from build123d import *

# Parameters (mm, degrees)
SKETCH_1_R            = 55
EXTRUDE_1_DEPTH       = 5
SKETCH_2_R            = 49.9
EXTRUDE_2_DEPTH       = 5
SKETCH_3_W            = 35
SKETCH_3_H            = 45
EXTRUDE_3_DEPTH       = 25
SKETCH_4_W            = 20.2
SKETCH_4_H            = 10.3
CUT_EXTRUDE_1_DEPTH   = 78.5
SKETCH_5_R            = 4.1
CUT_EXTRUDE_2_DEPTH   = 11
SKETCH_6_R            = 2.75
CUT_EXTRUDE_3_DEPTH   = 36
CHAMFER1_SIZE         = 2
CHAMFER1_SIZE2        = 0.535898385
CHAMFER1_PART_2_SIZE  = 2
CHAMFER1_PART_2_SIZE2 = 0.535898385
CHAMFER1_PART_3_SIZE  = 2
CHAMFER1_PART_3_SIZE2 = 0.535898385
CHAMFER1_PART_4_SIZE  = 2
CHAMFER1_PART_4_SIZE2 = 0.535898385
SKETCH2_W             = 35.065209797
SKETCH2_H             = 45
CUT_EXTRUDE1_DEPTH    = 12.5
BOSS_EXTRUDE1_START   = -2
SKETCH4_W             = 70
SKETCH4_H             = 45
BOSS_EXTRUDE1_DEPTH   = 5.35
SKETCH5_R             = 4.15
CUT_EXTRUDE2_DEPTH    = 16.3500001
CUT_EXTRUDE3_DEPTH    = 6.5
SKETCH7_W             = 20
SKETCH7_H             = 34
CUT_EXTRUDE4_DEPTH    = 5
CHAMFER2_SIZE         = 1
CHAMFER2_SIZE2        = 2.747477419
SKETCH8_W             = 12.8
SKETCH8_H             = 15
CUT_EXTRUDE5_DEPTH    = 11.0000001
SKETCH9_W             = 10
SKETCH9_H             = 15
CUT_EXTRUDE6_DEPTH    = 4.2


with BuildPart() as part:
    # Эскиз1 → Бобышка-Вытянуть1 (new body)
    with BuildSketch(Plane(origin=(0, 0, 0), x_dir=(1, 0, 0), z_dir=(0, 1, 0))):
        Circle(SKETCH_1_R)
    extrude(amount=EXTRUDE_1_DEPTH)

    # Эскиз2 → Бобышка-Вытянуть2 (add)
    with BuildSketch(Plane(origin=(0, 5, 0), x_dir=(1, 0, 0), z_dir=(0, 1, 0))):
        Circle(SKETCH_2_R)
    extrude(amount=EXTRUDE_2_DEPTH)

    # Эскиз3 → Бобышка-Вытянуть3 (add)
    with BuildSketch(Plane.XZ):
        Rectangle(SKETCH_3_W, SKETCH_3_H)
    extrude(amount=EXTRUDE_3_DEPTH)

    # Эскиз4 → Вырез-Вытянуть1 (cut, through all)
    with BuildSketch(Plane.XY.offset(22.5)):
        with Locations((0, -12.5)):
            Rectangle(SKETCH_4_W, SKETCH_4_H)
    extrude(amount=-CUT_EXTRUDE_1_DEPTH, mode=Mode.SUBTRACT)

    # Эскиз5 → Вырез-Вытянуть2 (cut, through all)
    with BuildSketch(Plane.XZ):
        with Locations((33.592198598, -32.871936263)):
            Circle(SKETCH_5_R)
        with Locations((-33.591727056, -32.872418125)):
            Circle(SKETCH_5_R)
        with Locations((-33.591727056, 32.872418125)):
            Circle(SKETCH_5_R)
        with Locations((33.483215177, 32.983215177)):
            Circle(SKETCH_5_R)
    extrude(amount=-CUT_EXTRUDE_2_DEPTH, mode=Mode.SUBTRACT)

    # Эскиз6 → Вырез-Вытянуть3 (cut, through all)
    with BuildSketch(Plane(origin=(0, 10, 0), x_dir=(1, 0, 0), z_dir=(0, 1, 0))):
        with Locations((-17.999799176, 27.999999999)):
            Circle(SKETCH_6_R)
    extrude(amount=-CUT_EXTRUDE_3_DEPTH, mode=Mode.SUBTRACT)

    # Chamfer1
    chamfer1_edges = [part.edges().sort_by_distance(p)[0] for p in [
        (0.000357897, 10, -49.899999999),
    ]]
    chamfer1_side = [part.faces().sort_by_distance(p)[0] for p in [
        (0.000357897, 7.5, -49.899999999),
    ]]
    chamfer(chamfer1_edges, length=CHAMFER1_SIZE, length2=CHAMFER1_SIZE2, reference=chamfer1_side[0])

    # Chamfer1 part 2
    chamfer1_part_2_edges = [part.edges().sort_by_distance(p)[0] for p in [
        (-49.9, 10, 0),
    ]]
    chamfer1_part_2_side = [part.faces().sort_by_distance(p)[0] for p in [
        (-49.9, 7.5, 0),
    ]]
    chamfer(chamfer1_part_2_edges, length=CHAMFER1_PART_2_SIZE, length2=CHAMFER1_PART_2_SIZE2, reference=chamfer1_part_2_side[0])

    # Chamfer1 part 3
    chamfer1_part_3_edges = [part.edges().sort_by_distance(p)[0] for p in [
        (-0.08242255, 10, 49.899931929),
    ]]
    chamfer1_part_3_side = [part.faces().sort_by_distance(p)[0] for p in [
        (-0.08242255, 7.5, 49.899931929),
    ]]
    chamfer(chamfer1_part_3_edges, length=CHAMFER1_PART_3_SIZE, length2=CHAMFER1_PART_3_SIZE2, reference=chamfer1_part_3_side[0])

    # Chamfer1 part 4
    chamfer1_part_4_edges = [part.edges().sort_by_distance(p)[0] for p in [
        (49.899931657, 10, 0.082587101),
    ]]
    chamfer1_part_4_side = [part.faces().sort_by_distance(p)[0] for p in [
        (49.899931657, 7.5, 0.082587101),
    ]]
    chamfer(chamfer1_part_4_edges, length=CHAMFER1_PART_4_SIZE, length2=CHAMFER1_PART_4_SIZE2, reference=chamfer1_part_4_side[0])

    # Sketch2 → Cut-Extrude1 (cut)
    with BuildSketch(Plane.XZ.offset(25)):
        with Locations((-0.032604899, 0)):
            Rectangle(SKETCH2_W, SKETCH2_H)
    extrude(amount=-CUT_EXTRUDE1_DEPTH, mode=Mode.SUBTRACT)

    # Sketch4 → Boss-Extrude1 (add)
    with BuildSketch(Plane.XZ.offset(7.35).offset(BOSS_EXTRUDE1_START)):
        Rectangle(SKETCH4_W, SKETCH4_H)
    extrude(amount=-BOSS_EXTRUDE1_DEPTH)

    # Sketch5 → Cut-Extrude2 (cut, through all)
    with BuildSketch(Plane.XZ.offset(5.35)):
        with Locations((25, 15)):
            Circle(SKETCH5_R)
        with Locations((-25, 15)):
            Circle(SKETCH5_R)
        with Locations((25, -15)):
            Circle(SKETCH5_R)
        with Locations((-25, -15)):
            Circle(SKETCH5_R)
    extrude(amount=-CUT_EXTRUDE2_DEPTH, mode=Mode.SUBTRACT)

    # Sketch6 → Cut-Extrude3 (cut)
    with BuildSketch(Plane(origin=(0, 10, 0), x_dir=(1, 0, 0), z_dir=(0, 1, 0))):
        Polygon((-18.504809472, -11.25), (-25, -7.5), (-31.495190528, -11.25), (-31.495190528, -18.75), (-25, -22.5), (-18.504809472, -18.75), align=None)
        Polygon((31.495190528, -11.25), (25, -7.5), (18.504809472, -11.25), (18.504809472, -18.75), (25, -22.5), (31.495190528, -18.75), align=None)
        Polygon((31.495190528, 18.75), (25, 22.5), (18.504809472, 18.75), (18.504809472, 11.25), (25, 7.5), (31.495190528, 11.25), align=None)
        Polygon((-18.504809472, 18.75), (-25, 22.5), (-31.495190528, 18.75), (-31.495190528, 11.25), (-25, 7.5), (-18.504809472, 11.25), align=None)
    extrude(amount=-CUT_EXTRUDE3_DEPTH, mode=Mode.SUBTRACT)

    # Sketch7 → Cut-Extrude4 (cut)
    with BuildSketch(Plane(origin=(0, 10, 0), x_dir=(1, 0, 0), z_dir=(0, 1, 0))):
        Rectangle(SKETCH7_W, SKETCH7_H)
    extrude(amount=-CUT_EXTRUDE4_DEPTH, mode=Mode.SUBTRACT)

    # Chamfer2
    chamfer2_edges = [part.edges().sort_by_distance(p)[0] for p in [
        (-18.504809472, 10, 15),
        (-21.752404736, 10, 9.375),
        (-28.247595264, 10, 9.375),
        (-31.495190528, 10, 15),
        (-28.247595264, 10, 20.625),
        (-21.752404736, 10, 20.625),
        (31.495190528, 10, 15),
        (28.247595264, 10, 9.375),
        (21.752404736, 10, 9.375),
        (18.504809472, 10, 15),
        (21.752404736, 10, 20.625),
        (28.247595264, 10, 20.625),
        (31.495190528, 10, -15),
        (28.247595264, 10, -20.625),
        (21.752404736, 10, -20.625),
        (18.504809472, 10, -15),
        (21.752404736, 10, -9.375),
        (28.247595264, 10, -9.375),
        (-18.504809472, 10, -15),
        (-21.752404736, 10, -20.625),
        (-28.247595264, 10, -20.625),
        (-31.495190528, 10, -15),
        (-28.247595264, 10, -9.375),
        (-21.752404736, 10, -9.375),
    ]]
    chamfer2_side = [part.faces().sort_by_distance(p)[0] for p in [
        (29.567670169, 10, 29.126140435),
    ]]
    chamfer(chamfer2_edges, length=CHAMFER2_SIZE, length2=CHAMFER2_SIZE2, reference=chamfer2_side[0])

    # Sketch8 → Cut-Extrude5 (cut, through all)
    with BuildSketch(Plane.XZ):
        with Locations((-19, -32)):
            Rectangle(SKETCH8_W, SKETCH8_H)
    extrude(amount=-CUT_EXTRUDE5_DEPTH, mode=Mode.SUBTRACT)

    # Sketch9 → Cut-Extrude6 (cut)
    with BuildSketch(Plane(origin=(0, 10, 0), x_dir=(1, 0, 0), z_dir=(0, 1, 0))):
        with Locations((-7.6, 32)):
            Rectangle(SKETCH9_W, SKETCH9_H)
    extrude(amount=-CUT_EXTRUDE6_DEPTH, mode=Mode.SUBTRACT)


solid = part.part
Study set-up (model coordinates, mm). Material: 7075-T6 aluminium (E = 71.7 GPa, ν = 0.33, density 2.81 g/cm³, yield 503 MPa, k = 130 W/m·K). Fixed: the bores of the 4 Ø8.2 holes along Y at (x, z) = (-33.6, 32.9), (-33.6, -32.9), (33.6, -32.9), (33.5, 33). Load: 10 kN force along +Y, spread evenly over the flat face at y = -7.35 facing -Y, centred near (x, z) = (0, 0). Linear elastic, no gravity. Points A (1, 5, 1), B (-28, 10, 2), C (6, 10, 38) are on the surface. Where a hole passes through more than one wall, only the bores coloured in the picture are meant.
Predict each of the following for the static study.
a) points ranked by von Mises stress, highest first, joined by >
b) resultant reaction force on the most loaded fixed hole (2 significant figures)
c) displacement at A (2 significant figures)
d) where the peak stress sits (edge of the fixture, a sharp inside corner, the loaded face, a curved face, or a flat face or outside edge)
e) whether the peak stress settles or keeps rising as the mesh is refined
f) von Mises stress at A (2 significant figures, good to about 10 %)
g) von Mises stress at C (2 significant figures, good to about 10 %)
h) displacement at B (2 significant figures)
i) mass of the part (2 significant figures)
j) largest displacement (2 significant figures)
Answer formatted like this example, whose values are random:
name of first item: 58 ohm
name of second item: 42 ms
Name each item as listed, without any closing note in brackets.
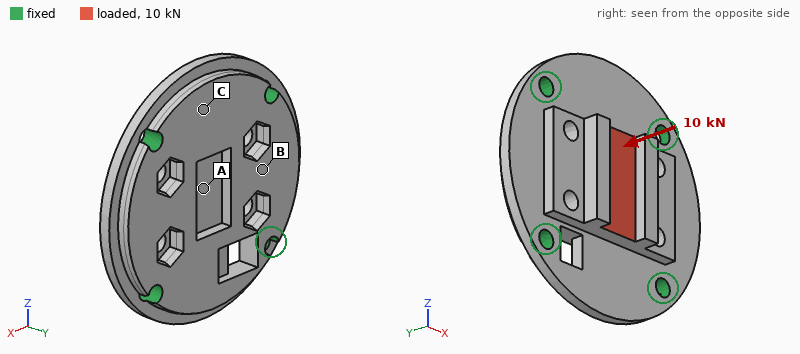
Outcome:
points ranked by von Mises stress, highest first, joined by >: A > C > B
resultant reaction force on the most loaded fixed hole: 3.3 kN
displacement at A: 44 µm
where the peak stress sits: edge of the fixture
whether the peak stress settles or keeps rising as the mesh is refined: keeps rising
von Mises stress at A: 31 MPa
von Mises stress at C: 19 MPa
displacement at B: 23 µm
mass of the part: 270 g
largest displacement: 45 µm
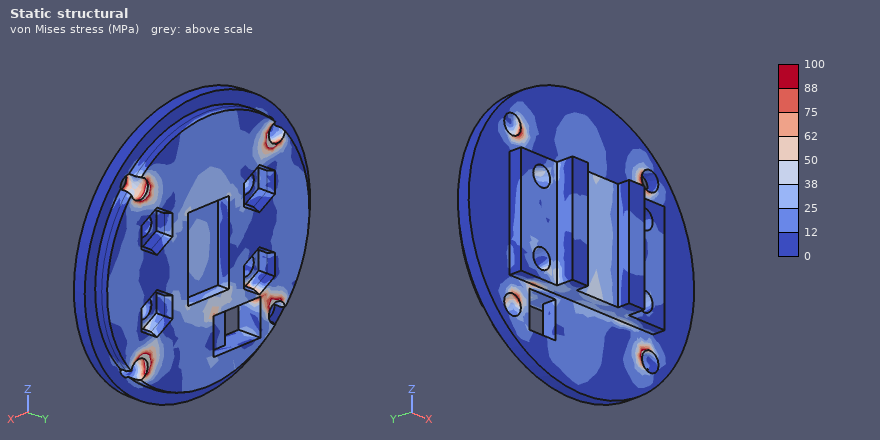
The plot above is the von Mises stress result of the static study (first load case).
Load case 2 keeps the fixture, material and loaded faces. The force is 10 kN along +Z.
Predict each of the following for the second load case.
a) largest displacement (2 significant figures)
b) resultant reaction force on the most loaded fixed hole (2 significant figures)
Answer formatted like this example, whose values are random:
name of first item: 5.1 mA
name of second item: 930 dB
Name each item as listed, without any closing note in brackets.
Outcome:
largest displacement: 21 µm
resultant reaction force on the most loaded fixed hole: 3.2 kN
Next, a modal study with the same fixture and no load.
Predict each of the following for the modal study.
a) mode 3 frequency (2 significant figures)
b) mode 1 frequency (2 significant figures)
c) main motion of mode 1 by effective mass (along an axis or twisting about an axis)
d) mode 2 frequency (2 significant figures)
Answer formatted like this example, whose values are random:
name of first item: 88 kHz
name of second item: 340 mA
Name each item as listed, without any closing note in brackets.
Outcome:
mode 3 frequency: 9900 Hz
mode 1 frequency: 7600 Hz
main motion of mode 1 by effective mass: along Y
mode 2 frequency: 9000 Hz
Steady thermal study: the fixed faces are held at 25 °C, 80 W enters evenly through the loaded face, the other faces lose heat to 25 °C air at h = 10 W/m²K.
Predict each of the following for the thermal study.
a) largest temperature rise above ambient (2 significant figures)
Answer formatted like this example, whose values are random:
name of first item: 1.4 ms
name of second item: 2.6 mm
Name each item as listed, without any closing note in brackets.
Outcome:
largest temperature rise above ambient: 20 K
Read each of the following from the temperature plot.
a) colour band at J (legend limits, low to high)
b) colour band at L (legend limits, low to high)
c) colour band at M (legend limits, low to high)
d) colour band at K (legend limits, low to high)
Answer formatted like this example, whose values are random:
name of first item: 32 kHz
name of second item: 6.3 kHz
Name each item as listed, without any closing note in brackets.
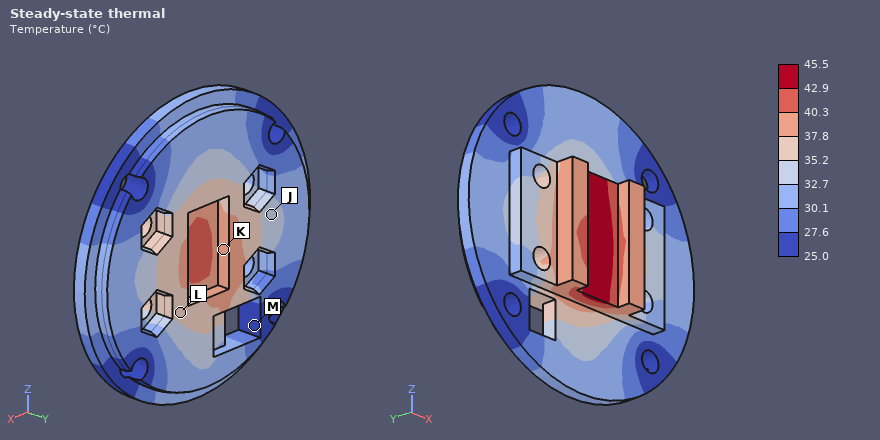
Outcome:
colour band at J: 32.7 to 35.2 °C
colour band at L: 35.2 to 37.8 °C
colour band at M: 25.0 to 27.6 °C
colour band at K: 37.8 to 40.3 °C
